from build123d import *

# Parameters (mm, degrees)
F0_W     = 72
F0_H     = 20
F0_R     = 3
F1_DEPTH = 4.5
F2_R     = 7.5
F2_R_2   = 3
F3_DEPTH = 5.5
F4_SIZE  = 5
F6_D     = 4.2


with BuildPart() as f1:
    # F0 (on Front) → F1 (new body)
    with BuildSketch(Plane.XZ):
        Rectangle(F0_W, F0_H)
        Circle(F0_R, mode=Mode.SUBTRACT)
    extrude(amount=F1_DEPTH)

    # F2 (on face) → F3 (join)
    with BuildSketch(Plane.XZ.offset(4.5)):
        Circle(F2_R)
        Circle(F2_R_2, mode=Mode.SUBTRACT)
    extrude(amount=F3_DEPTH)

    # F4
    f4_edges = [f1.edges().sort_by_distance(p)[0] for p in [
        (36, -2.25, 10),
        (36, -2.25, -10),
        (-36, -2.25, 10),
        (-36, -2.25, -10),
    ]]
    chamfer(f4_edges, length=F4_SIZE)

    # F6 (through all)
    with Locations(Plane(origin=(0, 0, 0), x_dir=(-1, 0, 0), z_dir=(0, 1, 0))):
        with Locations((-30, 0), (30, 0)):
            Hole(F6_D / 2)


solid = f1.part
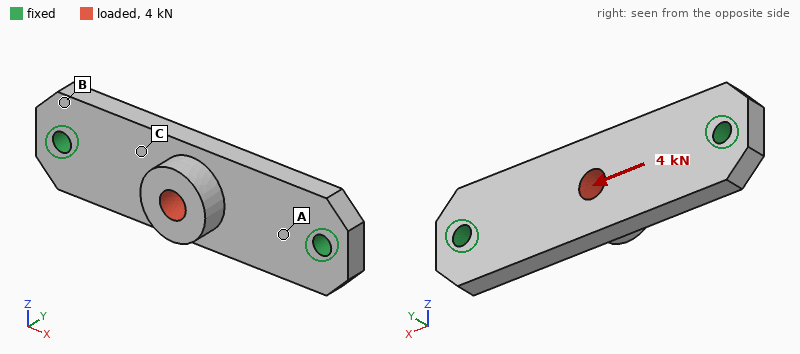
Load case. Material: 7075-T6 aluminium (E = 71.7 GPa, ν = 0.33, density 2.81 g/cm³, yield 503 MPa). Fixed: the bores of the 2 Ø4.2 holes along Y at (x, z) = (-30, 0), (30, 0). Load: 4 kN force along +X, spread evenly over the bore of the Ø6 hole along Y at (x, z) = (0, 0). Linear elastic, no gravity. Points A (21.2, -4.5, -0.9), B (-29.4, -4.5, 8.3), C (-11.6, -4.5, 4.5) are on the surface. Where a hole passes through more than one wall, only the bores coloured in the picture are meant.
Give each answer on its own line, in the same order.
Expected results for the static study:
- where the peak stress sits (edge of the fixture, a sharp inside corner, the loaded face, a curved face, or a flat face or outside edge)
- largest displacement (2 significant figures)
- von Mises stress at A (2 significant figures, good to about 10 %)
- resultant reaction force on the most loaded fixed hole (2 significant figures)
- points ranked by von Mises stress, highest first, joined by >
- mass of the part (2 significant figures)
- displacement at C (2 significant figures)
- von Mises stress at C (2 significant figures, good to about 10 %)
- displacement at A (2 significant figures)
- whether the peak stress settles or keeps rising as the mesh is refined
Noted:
edge of the fixture
32 µm
34 MPa
2.0 kN
C > A > B
19 g
16 µm
57 MPa
6.9 µm
keeps rising
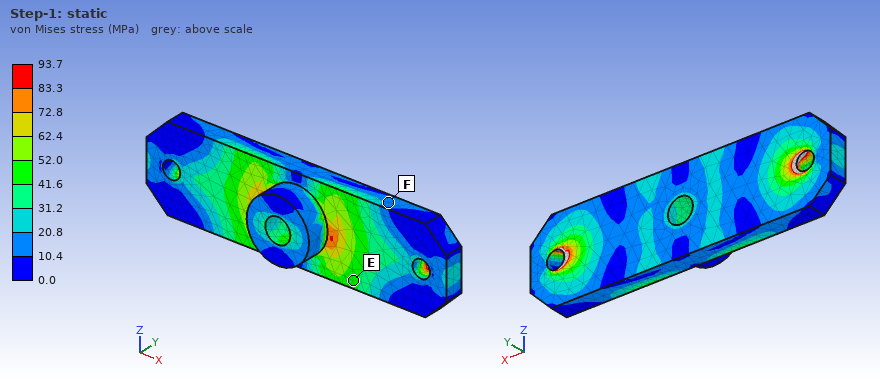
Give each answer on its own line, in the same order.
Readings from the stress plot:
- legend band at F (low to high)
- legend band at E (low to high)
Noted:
10.4 to 20.8 MPa
41.6 to 52.0 MPa
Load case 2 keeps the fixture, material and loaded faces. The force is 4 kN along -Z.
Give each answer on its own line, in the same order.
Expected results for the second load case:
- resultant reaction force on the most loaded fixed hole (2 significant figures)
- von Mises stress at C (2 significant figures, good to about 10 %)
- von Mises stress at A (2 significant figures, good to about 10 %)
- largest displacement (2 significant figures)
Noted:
2.0 kN
110 MPa
130 MPa
0.16 mm
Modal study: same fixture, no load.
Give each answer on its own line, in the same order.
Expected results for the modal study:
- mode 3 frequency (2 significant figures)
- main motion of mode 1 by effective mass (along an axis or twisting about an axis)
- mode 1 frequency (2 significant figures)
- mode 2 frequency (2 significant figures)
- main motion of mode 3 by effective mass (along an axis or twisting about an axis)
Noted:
13 kHz
along Y
6000 Hz
9100 Hz
along Z
